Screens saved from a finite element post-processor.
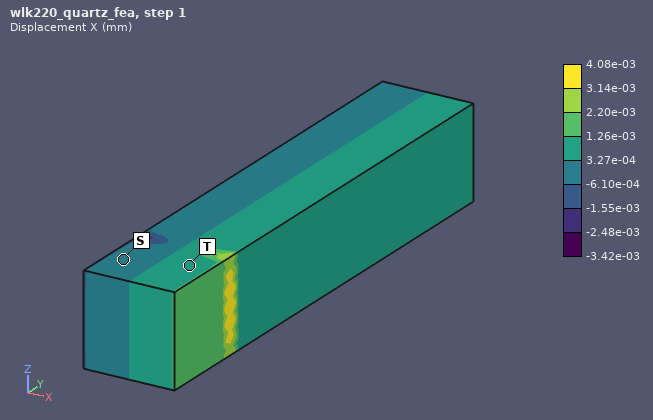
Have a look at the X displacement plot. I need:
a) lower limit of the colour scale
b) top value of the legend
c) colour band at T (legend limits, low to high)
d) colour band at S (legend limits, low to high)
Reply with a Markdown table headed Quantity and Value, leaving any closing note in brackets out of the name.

| Quantity | Value |
|---|---|
| lower limit of the colour scale | -3.42e-03 mm |
| top value of the legend | 4.08e-03 mm |
| colour band at T | 3.27e-04 to 1.26e-03 mm |
| colour band at S | -6.10e-04 to 3.27e-04 mm |
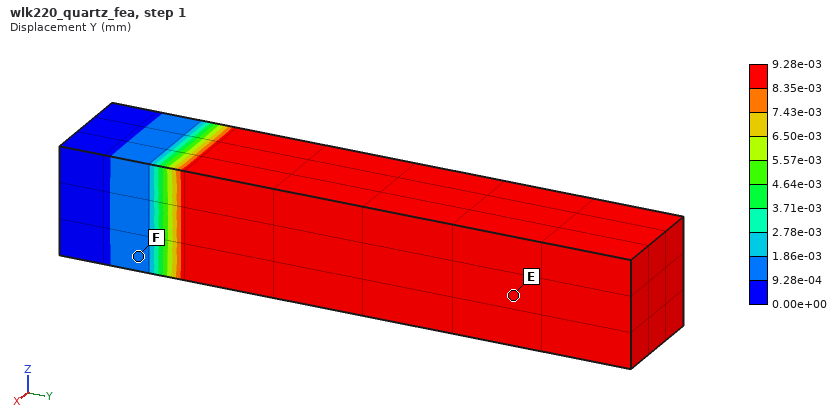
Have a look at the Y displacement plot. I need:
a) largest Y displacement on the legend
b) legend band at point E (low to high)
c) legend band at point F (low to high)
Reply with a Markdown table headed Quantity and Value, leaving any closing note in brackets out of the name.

| Quantity | Value |
|---|---|
| largest Y displacement on the legend | 9.28e-03 mm |
| legend band at point E | 8.35e-03 to 9.28e-03 mm |
| legend band at point F | 9.28e-04 to 1.86e-03 mm |
